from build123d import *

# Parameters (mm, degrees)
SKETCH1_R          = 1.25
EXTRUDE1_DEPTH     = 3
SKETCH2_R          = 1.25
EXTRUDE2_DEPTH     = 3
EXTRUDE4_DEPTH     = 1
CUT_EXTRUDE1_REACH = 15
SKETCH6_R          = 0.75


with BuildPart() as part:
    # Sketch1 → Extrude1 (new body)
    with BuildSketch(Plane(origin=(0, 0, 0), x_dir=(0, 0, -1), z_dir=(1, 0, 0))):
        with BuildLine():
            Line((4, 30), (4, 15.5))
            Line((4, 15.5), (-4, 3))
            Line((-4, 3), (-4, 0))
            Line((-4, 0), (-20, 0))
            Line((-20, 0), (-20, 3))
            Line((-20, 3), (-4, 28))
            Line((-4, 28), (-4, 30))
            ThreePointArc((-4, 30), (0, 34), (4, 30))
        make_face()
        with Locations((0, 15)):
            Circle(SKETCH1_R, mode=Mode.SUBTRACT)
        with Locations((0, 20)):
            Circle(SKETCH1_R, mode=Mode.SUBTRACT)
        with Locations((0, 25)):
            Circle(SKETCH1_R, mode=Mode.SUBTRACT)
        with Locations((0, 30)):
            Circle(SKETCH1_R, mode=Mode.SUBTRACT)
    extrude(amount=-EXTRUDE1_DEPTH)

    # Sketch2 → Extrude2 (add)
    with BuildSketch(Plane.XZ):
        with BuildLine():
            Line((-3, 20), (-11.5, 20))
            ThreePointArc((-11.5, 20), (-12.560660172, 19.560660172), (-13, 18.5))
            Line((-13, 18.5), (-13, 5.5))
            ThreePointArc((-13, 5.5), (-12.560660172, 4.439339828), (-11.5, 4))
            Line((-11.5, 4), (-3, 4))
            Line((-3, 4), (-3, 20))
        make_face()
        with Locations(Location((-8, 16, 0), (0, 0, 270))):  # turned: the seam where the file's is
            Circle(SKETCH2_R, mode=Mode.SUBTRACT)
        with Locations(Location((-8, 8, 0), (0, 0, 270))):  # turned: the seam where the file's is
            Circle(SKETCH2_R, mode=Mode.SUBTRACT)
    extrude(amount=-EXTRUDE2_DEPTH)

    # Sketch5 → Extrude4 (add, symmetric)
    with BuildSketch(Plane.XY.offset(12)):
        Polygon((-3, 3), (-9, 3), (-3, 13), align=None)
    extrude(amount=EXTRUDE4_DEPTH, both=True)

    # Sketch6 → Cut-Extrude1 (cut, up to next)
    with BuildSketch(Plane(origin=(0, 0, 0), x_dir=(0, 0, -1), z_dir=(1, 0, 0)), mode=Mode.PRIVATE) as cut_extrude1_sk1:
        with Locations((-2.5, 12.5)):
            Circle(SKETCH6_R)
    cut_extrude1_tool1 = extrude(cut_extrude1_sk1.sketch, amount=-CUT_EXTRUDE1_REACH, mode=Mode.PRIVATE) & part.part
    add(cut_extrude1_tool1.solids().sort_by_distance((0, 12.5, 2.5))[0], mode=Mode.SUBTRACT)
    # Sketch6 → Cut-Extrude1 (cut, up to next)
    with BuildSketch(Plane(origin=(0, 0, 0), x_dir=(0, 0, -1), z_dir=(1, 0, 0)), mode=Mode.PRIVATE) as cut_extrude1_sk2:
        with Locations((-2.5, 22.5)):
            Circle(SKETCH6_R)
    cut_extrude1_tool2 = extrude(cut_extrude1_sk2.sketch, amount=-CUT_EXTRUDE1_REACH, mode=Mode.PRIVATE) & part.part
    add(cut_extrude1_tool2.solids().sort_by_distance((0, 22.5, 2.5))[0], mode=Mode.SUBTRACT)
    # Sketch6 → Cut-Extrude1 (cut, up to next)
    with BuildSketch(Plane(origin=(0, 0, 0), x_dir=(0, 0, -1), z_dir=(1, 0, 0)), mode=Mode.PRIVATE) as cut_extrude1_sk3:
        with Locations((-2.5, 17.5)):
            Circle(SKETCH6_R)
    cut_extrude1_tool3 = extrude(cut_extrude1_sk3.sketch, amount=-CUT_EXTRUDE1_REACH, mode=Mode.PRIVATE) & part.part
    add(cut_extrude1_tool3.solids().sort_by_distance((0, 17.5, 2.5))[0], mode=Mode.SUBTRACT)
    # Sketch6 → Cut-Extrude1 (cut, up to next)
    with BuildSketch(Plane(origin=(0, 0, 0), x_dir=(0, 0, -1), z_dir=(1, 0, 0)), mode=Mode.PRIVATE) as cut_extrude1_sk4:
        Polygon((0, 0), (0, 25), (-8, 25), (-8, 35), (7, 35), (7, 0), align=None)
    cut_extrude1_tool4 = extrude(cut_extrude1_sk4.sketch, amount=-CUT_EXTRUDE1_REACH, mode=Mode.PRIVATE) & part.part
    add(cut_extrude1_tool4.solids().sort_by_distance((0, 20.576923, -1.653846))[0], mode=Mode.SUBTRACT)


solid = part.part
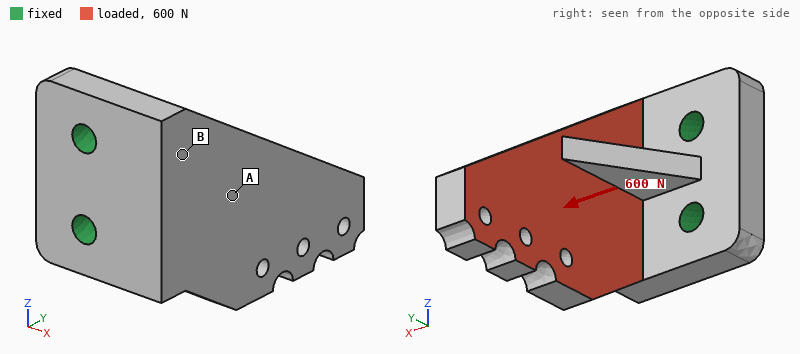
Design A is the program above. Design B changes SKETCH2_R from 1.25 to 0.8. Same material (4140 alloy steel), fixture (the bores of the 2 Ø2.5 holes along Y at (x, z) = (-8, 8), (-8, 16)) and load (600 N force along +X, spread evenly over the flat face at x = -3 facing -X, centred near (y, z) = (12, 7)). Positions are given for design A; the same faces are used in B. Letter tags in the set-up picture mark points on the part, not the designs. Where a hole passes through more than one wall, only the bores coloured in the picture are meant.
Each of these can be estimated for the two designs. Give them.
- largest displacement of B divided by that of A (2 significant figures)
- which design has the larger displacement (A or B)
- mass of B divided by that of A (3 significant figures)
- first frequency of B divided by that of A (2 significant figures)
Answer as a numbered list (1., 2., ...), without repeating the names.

1. 1.1
2. B
3. 1.01
4. 0.94
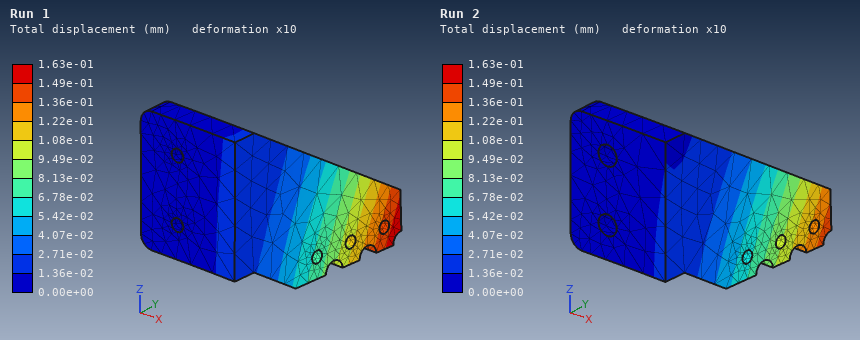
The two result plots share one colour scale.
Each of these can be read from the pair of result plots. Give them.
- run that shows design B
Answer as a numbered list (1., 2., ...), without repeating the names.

1. Run 1
